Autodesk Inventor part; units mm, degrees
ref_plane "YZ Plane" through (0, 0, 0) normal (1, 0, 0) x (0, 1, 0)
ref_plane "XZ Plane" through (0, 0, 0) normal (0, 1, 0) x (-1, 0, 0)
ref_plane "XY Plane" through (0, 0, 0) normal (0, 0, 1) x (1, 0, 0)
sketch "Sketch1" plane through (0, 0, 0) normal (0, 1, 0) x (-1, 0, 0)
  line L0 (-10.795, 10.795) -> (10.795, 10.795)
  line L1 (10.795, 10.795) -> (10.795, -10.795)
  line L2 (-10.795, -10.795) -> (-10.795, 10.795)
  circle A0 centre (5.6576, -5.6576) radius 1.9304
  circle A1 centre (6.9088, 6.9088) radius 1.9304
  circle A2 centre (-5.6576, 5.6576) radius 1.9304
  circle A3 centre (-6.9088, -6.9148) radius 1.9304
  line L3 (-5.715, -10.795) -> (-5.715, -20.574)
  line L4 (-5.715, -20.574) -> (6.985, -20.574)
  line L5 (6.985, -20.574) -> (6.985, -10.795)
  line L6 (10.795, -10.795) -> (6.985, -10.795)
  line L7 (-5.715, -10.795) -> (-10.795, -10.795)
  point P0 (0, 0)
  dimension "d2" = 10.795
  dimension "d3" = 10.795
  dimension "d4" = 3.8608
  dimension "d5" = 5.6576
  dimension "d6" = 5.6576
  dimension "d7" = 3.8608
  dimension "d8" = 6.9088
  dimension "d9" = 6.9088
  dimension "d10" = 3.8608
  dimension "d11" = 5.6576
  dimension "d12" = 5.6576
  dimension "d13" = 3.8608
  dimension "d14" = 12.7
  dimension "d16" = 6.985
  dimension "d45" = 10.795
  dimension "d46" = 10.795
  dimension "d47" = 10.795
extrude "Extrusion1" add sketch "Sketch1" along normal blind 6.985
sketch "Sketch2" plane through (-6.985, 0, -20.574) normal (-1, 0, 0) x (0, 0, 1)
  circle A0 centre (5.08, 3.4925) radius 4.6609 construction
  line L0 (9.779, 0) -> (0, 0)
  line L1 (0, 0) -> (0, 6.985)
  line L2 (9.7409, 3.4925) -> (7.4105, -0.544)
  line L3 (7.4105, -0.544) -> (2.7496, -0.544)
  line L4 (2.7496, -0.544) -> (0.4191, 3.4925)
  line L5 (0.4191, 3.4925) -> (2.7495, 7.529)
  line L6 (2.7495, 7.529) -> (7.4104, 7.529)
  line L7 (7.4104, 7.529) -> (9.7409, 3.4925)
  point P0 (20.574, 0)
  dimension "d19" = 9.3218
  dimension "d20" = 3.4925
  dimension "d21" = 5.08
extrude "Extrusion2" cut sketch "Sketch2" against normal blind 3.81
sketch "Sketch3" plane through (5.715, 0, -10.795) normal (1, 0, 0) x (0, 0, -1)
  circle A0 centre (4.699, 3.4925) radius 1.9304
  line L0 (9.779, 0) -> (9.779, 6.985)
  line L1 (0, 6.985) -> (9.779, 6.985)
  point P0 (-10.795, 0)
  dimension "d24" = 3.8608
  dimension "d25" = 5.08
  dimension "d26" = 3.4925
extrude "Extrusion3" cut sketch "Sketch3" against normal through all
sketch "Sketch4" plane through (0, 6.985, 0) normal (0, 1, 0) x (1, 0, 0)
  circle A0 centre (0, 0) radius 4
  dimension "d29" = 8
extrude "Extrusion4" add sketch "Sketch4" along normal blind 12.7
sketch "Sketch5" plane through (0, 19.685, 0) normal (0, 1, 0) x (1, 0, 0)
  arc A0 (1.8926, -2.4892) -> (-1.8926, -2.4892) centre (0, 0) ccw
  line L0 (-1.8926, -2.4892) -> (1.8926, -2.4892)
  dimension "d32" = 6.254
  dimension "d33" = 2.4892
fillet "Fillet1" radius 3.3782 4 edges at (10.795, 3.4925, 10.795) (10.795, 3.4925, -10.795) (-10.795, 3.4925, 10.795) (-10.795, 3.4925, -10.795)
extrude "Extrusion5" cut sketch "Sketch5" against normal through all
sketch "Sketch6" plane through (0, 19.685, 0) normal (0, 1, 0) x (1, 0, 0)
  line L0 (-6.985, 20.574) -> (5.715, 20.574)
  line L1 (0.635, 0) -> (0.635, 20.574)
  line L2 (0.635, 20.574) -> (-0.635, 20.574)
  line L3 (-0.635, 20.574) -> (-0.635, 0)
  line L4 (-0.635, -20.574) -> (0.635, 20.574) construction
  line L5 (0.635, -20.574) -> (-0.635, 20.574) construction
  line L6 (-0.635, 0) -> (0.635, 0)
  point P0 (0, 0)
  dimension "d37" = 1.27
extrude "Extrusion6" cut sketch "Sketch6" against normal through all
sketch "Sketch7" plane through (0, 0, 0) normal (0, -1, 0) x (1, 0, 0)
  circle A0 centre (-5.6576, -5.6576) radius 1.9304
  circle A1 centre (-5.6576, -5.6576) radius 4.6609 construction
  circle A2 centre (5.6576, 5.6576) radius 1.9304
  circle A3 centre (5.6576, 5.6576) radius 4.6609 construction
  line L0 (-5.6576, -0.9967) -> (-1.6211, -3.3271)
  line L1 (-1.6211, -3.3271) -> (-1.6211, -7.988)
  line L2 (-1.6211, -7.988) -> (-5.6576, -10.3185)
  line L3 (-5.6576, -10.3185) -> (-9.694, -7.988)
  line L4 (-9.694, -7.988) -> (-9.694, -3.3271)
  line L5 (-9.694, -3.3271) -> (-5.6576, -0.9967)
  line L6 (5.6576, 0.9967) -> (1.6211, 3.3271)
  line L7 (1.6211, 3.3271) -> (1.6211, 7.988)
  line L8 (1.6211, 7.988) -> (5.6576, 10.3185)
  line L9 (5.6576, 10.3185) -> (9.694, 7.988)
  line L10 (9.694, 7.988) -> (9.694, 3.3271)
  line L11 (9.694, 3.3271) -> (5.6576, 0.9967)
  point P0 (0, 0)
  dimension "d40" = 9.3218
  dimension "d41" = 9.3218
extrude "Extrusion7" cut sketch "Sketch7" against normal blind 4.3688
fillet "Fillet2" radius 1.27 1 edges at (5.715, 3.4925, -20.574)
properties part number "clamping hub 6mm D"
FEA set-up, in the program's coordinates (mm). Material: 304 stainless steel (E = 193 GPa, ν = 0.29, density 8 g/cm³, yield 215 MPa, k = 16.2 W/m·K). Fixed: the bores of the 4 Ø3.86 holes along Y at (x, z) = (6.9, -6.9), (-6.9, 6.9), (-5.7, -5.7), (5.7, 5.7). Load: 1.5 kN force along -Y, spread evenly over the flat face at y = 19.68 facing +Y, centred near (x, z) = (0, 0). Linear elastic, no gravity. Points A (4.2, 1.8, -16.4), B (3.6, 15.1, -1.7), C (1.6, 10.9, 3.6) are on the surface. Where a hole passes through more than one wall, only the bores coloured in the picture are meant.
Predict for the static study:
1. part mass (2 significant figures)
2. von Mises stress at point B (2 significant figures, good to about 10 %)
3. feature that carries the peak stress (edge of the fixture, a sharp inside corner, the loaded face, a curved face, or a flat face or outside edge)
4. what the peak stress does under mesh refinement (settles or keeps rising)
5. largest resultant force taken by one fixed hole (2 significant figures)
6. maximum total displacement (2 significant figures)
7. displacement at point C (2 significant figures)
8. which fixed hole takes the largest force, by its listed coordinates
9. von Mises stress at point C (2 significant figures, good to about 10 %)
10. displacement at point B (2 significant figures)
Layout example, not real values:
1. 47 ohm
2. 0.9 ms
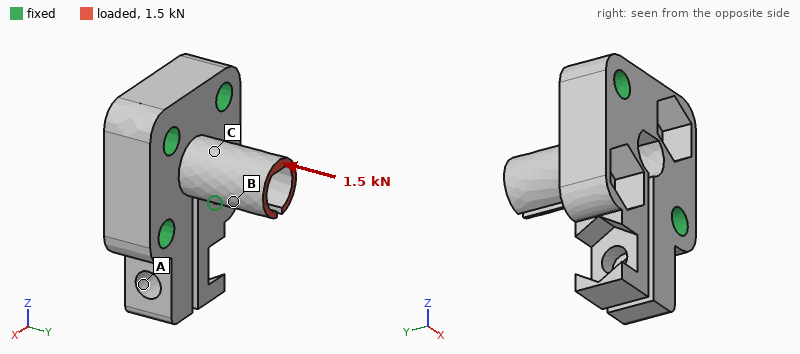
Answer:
1. 24 g
2. 75 MPa
3. edge of the fixture
4. keeps rising
5. 480 N
6. 7.3 µm
7. 3.0 µm
8. (-6.9, 6.9)
9. 68 MPa
10. 4.5 µm
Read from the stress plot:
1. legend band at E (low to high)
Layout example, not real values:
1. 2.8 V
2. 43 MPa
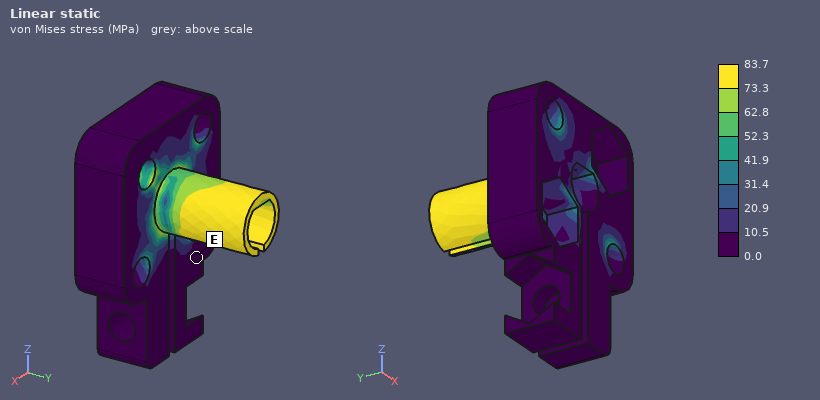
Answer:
1. 0.0 to 10.5 MPa
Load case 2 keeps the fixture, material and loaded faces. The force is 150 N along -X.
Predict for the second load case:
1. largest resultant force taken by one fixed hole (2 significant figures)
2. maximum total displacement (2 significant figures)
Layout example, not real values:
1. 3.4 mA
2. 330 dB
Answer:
1. 150 N
2. 33 µm
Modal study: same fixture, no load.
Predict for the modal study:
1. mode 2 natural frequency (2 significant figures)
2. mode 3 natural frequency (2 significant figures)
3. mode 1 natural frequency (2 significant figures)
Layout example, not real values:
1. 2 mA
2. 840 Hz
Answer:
1. 13 kHz
2. 15 kHz
3. 11 kHz
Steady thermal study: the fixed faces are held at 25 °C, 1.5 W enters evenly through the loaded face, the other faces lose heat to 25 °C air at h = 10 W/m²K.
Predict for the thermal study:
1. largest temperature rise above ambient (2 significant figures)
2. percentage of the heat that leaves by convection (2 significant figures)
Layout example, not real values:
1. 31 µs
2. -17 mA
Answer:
1. 60 K
2. 13 %
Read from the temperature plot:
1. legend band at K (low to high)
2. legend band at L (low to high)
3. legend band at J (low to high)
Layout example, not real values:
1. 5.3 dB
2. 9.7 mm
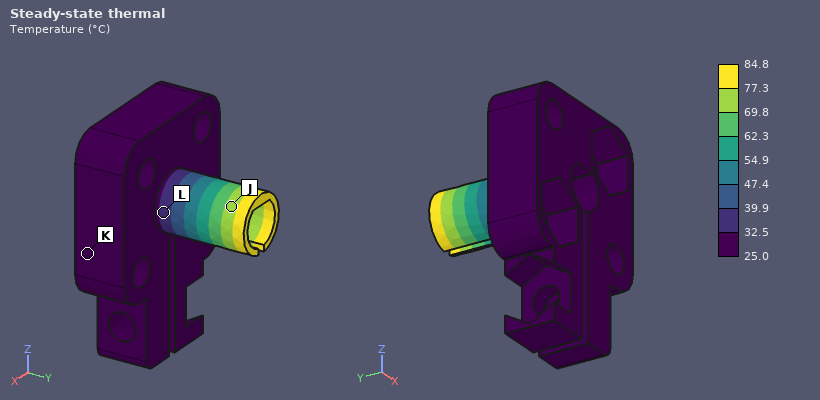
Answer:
1. 25.0 to 32.5 °C
2. 32.5 to 39.9 °C
3. 69.8 to 77.3 °C
